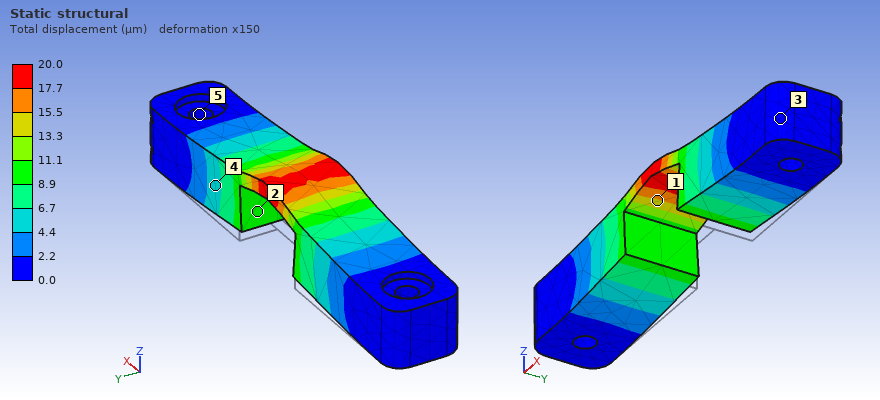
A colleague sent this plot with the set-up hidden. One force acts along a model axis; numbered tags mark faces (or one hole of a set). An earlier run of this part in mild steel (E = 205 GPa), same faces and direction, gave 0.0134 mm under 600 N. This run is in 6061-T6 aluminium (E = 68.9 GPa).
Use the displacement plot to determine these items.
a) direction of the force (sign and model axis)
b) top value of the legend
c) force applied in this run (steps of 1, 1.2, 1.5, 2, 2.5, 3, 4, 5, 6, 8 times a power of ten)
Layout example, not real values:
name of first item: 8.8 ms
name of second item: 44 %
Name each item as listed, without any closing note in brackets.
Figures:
direction of the force: +Z
top value of the legend: 20.0 µm
force applied in this run: 300 N
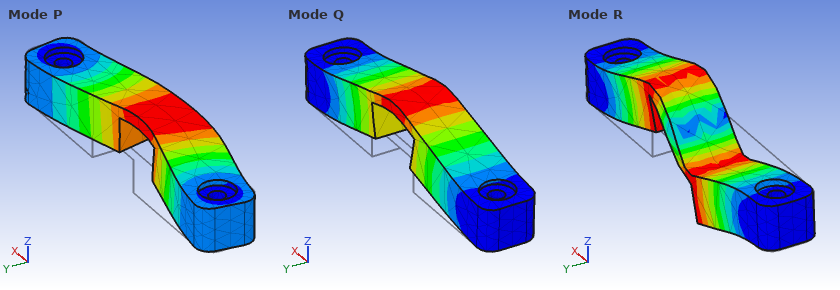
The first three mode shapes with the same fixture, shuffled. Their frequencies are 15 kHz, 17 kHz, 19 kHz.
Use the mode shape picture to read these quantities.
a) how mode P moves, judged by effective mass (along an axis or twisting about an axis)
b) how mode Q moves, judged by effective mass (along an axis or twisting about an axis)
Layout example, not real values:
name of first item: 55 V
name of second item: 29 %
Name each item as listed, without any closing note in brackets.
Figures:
how mode P moves, judged by effective mass: along Y
how mode Q moves, judged by effective mass: along Z
